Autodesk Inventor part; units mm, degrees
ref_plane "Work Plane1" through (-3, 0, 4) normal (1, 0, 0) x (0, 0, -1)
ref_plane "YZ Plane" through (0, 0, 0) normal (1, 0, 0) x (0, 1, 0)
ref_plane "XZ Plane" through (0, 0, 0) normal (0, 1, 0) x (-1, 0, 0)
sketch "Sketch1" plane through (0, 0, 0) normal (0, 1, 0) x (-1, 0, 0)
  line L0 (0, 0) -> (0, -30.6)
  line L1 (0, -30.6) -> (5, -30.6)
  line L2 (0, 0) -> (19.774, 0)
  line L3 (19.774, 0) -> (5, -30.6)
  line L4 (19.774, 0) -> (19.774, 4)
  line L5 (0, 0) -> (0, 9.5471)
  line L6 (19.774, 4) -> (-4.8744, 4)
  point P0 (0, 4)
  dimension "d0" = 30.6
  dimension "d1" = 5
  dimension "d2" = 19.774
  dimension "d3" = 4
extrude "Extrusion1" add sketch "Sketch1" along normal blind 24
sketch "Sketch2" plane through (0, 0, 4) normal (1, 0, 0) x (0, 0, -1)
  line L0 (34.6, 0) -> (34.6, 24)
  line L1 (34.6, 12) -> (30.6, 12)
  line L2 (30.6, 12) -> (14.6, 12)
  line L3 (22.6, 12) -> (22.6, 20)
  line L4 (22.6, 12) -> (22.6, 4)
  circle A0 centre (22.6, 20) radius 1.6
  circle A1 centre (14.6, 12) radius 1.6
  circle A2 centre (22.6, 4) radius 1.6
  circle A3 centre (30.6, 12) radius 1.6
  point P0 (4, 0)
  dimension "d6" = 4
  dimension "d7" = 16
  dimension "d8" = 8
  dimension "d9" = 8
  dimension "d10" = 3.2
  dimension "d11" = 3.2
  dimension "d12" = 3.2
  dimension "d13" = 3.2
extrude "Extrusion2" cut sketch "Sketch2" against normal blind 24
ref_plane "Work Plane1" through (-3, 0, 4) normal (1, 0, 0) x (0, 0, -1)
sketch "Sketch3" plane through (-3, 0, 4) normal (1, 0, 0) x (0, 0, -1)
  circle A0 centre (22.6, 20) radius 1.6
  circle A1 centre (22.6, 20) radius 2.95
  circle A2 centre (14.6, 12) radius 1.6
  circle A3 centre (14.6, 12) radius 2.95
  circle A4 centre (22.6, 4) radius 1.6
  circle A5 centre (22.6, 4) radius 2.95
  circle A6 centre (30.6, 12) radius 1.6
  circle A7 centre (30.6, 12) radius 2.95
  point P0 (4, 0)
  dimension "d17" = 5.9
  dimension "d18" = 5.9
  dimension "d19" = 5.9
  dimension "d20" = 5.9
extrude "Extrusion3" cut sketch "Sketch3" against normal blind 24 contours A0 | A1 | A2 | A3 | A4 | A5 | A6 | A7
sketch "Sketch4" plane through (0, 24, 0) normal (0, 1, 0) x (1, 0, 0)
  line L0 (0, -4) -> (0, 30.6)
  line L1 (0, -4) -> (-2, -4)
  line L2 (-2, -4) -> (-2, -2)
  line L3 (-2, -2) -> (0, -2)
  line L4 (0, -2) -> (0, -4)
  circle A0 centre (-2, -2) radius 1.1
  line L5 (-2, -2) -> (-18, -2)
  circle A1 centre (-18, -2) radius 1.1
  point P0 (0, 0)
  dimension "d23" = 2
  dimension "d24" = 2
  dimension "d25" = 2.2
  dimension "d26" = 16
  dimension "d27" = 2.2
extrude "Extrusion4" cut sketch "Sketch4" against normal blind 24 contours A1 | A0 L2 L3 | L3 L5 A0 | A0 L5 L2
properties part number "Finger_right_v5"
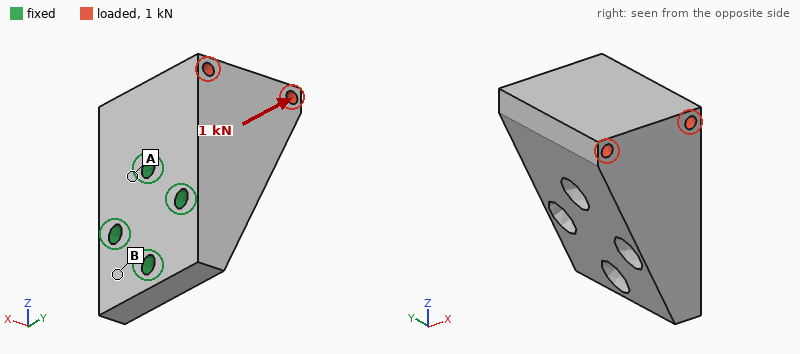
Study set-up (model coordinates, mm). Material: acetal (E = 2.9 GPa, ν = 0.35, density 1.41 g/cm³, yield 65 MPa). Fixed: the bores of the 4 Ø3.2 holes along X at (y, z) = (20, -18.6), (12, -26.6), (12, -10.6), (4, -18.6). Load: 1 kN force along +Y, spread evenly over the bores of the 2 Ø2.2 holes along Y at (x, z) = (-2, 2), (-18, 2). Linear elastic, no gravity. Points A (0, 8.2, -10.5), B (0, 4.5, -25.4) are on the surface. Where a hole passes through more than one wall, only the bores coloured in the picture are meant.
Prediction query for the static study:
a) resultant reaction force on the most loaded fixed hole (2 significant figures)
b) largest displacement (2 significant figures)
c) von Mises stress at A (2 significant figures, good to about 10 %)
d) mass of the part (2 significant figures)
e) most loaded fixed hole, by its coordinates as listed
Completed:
910 N
0.35 mm
17 MPa
14 g
(12, -10.6)
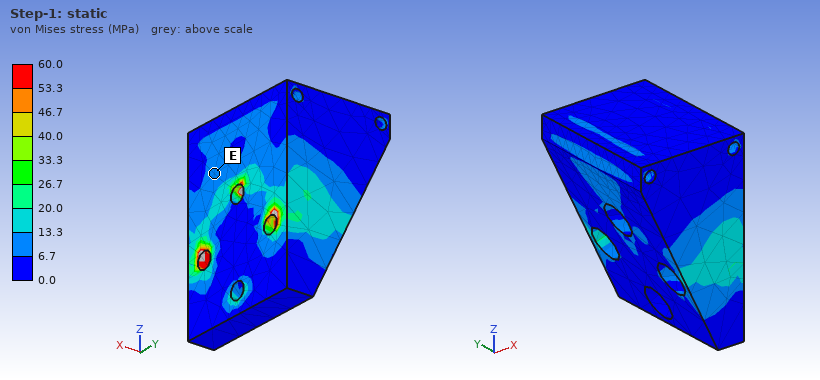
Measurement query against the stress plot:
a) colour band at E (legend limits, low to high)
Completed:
6.7 to 13.3 MPa
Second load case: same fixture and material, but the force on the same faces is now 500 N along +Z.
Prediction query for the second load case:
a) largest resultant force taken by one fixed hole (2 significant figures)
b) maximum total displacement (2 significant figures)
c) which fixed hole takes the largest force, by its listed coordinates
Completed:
310 N
0.15 mm
(12, -10.6)
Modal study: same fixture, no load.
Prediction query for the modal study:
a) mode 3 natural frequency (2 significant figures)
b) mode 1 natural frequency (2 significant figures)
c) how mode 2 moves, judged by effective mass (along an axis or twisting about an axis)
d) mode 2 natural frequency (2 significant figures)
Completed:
6000 Hz
3000 Hz
along Y
3900 Hz
